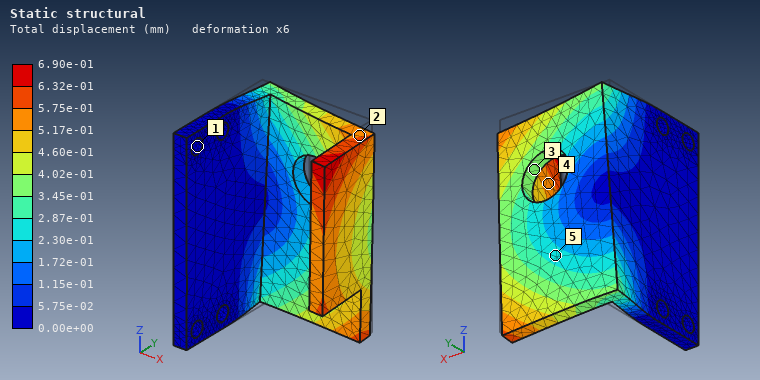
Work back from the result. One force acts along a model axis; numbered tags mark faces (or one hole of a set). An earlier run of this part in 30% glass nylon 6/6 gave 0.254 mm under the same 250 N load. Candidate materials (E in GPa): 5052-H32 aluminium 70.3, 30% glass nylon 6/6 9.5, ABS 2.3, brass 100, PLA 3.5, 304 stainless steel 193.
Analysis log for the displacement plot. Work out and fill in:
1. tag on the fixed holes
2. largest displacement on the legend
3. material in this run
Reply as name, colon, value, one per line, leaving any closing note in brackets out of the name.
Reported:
tag on the fixed holes: 1
largest displacement on the legend: 6.90e-01 mm
material in this run: PLA
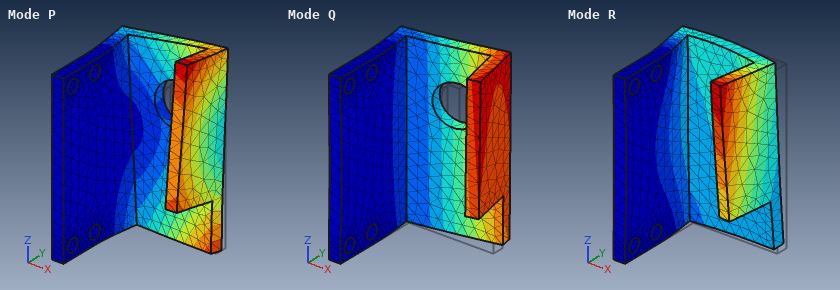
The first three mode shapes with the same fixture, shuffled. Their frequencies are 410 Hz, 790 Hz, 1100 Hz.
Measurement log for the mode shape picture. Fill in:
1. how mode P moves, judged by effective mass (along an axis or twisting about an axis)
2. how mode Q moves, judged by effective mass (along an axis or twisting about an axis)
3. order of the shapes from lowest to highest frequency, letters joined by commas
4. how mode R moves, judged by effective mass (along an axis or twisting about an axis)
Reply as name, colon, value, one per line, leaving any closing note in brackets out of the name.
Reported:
how mode P moves, judged by effective mass: along Z
how mode Q moves, judged by effective mass: along Y
order of the shapes from lowest to highest frequency, letters joined by commas: Q, P, R
how mode R moves, judged by effective mass: along X
